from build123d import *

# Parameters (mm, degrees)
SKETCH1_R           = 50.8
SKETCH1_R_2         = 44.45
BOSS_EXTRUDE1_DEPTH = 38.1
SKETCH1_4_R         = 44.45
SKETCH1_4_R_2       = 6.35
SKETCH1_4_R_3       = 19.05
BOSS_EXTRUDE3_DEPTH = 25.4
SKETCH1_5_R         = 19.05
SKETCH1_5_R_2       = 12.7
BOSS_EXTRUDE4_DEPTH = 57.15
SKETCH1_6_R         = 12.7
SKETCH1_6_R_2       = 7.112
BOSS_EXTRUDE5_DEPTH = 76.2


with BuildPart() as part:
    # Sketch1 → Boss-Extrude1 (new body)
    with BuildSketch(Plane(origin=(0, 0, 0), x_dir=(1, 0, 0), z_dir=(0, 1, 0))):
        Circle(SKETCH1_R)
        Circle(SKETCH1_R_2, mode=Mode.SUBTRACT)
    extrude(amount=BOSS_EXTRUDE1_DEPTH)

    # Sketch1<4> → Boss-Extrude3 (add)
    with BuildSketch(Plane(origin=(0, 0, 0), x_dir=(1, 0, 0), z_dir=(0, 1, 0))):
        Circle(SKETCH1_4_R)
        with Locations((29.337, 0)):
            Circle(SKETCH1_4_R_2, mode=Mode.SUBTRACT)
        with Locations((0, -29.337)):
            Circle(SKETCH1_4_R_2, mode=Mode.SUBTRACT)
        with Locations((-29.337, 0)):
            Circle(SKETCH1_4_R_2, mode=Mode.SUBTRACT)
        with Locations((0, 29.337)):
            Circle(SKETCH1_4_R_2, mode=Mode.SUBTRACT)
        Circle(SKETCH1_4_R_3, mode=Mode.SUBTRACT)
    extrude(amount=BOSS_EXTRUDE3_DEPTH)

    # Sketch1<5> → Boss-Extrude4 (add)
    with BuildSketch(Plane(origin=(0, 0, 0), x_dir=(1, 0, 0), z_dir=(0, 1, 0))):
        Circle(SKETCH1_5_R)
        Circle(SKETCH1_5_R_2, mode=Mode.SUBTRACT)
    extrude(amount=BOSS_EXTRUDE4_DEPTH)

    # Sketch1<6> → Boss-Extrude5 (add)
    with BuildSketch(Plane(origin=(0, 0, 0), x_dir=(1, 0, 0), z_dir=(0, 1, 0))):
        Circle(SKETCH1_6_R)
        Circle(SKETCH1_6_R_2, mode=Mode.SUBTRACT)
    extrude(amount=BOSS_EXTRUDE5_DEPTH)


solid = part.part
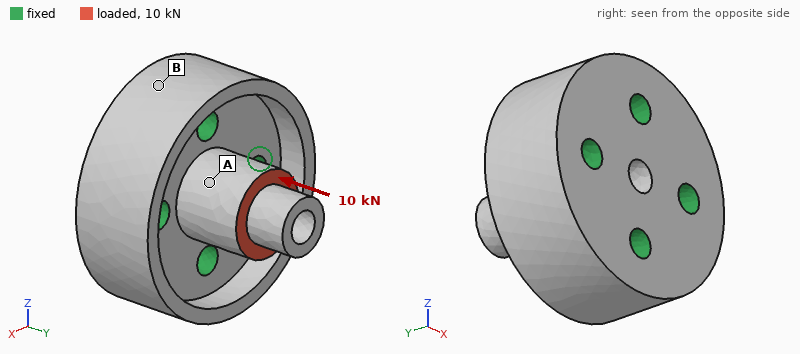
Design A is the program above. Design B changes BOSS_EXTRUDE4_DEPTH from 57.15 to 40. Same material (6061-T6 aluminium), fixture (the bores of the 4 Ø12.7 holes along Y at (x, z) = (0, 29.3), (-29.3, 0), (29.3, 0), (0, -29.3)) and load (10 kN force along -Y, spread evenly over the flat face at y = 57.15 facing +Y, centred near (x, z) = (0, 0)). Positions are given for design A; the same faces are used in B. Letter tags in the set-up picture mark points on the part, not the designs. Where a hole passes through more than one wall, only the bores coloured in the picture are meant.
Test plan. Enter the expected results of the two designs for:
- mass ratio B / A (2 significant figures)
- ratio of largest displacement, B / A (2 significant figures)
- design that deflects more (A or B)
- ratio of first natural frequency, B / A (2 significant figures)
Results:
0.96
0.70
A
0.90
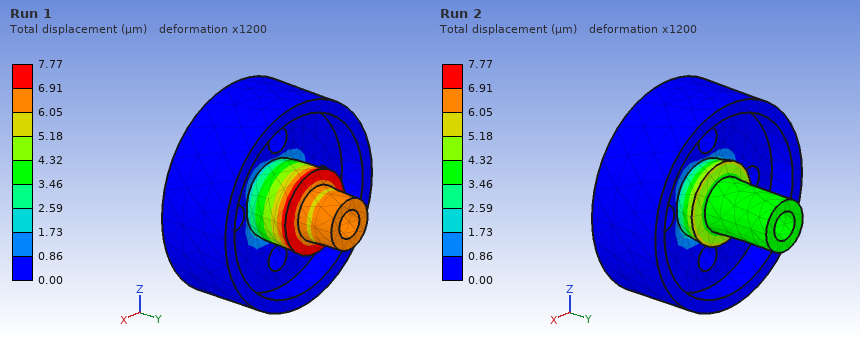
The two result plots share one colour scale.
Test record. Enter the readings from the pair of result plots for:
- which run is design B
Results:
Run 2
